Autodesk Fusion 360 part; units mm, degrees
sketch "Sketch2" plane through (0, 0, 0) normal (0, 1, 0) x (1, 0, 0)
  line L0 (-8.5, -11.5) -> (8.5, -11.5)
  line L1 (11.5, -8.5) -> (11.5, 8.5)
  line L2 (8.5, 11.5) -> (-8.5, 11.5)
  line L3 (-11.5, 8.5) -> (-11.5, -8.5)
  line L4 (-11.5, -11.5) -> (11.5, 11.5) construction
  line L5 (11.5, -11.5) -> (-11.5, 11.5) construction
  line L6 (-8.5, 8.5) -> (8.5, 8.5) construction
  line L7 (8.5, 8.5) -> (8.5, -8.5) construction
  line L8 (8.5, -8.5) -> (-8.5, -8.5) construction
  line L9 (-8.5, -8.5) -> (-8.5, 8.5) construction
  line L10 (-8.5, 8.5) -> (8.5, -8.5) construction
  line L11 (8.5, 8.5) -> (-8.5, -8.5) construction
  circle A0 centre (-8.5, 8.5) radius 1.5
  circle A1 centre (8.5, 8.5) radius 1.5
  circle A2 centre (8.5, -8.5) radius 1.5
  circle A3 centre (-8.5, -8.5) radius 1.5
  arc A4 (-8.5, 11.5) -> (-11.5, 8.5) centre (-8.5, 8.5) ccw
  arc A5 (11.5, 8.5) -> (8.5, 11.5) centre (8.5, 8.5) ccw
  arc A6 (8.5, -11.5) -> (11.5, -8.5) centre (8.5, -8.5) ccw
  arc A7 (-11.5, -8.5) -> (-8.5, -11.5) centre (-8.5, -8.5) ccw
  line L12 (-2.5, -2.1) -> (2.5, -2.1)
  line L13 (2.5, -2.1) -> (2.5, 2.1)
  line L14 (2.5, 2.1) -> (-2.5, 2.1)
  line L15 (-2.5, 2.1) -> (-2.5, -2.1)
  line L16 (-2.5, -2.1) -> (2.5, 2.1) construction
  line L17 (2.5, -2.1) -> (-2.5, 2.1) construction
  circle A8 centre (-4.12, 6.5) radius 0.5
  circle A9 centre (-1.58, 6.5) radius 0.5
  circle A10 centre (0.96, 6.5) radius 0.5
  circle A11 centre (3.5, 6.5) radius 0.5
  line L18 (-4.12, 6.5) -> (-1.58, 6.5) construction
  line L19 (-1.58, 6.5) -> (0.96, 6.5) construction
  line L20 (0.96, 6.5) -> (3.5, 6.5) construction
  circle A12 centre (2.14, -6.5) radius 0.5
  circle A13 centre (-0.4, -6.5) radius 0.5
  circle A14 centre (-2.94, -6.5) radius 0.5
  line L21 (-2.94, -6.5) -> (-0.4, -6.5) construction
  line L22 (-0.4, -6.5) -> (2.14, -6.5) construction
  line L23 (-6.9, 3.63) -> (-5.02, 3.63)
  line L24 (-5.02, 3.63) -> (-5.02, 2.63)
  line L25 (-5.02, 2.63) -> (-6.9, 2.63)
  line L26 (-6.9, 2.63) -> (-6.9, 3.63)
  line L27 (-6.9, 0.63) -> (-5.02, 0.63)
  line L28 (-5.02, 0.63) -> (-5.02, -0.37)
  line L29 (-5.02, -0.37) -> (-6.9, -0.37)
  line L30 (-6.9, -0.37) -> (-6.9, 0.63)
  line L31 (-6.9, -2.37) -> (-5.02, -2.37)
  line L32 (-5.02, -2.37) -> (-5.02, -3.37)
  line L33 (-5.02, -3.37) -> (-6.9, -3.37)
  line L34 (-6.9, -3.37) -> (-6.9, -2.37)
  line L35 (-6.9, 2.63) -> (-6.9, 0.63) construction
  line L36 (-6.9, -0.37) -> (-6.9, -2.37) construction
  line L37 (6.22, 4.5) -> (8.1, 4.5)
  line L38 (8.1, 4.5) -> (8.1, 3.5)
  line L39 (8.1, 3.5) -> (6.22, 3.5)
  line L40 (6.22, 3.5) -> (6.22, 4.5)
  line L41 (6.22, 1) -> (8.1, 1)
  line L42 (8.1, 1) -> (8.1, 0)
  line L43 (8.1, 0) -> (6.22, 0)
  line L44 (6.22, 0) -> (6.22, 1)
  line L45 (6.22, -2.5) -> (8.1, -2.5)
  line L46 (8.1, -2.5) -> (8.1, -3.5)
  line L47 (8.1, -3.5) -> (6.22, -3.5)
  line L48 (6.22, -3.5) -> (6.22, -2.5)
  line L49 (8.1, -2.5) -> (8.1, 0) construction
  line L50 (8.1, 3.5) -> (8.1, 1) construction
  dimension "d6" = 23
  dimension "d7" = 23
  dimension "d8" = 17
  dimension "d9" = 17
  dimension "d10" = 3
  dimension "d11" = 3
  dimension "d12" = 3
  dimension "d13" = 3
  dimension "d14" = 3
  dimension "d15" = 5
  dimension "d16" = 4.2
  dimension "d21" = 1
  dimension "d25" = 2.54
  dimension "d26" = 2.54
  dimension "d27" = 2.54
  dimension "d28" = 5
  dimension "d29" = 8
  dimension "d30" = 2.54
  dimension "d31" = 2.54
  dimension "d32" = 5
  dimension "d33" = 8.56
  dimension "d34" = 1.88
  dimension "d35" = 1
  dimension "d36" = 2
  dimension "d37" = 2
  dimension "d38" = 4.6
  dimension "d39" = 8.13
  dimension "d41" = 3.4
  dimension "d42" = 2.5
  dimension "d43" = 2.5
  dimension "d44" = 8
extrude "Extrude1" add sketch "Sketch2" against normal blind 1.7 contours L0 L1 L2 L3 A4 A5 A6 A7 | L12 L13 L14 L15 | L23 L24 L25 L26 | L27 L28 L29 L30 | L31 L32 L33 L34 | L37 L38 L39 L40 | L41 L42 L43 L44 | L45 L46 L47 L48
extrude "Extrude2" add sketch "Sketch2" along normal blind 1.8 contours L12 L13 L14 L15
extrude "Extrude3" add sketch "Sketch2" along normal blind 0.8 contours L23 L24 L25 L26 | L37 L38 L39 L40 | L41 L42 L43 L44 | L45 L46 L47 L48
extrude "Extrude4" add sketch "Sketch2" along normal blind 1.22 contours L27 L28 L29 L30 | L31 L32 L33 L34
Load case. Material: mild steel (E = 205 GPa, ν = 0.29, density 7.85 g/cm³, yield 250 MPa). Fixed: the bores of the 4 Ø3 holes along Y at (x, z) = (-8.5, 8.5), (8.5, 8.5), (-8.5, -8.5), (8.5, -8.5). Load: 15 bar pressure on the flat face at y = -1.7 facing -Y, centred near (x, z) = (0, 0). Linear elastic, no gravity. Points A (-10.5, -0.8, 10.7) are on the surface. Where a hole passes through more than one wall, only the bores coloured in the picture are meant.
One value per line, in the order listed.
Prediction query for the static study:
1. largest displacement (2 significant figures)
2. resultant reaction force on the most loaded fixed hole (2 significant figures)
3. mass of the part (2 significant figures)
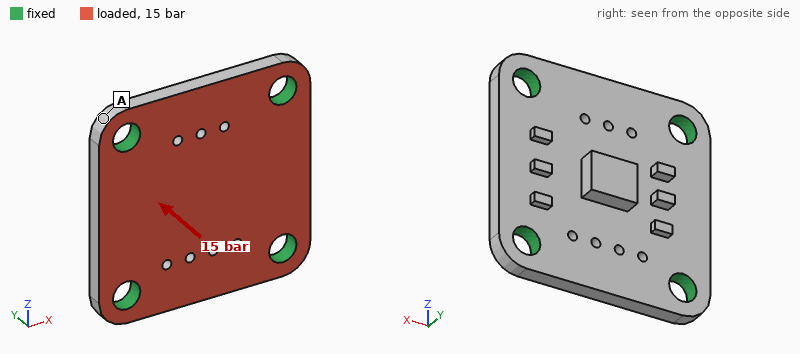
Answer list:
5.7 µm
180 N
6.9 g
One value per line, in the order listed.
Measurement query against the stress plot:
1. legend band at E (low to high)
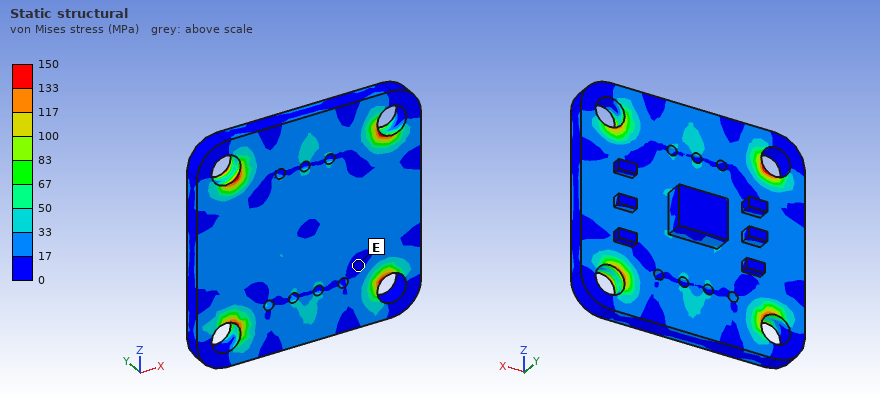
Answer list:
0 to 17 MPa
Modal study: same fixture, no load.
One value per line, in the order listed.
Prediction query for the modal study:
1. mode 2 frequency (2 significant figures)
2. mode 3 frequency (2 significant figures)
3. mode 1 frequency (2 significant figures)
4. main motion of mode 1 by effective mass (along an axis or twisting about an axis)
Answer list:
38 kHz
39 kHz
24 kHz
along Y
